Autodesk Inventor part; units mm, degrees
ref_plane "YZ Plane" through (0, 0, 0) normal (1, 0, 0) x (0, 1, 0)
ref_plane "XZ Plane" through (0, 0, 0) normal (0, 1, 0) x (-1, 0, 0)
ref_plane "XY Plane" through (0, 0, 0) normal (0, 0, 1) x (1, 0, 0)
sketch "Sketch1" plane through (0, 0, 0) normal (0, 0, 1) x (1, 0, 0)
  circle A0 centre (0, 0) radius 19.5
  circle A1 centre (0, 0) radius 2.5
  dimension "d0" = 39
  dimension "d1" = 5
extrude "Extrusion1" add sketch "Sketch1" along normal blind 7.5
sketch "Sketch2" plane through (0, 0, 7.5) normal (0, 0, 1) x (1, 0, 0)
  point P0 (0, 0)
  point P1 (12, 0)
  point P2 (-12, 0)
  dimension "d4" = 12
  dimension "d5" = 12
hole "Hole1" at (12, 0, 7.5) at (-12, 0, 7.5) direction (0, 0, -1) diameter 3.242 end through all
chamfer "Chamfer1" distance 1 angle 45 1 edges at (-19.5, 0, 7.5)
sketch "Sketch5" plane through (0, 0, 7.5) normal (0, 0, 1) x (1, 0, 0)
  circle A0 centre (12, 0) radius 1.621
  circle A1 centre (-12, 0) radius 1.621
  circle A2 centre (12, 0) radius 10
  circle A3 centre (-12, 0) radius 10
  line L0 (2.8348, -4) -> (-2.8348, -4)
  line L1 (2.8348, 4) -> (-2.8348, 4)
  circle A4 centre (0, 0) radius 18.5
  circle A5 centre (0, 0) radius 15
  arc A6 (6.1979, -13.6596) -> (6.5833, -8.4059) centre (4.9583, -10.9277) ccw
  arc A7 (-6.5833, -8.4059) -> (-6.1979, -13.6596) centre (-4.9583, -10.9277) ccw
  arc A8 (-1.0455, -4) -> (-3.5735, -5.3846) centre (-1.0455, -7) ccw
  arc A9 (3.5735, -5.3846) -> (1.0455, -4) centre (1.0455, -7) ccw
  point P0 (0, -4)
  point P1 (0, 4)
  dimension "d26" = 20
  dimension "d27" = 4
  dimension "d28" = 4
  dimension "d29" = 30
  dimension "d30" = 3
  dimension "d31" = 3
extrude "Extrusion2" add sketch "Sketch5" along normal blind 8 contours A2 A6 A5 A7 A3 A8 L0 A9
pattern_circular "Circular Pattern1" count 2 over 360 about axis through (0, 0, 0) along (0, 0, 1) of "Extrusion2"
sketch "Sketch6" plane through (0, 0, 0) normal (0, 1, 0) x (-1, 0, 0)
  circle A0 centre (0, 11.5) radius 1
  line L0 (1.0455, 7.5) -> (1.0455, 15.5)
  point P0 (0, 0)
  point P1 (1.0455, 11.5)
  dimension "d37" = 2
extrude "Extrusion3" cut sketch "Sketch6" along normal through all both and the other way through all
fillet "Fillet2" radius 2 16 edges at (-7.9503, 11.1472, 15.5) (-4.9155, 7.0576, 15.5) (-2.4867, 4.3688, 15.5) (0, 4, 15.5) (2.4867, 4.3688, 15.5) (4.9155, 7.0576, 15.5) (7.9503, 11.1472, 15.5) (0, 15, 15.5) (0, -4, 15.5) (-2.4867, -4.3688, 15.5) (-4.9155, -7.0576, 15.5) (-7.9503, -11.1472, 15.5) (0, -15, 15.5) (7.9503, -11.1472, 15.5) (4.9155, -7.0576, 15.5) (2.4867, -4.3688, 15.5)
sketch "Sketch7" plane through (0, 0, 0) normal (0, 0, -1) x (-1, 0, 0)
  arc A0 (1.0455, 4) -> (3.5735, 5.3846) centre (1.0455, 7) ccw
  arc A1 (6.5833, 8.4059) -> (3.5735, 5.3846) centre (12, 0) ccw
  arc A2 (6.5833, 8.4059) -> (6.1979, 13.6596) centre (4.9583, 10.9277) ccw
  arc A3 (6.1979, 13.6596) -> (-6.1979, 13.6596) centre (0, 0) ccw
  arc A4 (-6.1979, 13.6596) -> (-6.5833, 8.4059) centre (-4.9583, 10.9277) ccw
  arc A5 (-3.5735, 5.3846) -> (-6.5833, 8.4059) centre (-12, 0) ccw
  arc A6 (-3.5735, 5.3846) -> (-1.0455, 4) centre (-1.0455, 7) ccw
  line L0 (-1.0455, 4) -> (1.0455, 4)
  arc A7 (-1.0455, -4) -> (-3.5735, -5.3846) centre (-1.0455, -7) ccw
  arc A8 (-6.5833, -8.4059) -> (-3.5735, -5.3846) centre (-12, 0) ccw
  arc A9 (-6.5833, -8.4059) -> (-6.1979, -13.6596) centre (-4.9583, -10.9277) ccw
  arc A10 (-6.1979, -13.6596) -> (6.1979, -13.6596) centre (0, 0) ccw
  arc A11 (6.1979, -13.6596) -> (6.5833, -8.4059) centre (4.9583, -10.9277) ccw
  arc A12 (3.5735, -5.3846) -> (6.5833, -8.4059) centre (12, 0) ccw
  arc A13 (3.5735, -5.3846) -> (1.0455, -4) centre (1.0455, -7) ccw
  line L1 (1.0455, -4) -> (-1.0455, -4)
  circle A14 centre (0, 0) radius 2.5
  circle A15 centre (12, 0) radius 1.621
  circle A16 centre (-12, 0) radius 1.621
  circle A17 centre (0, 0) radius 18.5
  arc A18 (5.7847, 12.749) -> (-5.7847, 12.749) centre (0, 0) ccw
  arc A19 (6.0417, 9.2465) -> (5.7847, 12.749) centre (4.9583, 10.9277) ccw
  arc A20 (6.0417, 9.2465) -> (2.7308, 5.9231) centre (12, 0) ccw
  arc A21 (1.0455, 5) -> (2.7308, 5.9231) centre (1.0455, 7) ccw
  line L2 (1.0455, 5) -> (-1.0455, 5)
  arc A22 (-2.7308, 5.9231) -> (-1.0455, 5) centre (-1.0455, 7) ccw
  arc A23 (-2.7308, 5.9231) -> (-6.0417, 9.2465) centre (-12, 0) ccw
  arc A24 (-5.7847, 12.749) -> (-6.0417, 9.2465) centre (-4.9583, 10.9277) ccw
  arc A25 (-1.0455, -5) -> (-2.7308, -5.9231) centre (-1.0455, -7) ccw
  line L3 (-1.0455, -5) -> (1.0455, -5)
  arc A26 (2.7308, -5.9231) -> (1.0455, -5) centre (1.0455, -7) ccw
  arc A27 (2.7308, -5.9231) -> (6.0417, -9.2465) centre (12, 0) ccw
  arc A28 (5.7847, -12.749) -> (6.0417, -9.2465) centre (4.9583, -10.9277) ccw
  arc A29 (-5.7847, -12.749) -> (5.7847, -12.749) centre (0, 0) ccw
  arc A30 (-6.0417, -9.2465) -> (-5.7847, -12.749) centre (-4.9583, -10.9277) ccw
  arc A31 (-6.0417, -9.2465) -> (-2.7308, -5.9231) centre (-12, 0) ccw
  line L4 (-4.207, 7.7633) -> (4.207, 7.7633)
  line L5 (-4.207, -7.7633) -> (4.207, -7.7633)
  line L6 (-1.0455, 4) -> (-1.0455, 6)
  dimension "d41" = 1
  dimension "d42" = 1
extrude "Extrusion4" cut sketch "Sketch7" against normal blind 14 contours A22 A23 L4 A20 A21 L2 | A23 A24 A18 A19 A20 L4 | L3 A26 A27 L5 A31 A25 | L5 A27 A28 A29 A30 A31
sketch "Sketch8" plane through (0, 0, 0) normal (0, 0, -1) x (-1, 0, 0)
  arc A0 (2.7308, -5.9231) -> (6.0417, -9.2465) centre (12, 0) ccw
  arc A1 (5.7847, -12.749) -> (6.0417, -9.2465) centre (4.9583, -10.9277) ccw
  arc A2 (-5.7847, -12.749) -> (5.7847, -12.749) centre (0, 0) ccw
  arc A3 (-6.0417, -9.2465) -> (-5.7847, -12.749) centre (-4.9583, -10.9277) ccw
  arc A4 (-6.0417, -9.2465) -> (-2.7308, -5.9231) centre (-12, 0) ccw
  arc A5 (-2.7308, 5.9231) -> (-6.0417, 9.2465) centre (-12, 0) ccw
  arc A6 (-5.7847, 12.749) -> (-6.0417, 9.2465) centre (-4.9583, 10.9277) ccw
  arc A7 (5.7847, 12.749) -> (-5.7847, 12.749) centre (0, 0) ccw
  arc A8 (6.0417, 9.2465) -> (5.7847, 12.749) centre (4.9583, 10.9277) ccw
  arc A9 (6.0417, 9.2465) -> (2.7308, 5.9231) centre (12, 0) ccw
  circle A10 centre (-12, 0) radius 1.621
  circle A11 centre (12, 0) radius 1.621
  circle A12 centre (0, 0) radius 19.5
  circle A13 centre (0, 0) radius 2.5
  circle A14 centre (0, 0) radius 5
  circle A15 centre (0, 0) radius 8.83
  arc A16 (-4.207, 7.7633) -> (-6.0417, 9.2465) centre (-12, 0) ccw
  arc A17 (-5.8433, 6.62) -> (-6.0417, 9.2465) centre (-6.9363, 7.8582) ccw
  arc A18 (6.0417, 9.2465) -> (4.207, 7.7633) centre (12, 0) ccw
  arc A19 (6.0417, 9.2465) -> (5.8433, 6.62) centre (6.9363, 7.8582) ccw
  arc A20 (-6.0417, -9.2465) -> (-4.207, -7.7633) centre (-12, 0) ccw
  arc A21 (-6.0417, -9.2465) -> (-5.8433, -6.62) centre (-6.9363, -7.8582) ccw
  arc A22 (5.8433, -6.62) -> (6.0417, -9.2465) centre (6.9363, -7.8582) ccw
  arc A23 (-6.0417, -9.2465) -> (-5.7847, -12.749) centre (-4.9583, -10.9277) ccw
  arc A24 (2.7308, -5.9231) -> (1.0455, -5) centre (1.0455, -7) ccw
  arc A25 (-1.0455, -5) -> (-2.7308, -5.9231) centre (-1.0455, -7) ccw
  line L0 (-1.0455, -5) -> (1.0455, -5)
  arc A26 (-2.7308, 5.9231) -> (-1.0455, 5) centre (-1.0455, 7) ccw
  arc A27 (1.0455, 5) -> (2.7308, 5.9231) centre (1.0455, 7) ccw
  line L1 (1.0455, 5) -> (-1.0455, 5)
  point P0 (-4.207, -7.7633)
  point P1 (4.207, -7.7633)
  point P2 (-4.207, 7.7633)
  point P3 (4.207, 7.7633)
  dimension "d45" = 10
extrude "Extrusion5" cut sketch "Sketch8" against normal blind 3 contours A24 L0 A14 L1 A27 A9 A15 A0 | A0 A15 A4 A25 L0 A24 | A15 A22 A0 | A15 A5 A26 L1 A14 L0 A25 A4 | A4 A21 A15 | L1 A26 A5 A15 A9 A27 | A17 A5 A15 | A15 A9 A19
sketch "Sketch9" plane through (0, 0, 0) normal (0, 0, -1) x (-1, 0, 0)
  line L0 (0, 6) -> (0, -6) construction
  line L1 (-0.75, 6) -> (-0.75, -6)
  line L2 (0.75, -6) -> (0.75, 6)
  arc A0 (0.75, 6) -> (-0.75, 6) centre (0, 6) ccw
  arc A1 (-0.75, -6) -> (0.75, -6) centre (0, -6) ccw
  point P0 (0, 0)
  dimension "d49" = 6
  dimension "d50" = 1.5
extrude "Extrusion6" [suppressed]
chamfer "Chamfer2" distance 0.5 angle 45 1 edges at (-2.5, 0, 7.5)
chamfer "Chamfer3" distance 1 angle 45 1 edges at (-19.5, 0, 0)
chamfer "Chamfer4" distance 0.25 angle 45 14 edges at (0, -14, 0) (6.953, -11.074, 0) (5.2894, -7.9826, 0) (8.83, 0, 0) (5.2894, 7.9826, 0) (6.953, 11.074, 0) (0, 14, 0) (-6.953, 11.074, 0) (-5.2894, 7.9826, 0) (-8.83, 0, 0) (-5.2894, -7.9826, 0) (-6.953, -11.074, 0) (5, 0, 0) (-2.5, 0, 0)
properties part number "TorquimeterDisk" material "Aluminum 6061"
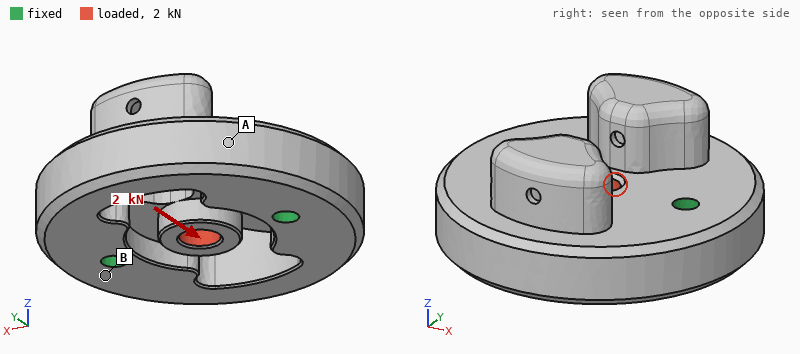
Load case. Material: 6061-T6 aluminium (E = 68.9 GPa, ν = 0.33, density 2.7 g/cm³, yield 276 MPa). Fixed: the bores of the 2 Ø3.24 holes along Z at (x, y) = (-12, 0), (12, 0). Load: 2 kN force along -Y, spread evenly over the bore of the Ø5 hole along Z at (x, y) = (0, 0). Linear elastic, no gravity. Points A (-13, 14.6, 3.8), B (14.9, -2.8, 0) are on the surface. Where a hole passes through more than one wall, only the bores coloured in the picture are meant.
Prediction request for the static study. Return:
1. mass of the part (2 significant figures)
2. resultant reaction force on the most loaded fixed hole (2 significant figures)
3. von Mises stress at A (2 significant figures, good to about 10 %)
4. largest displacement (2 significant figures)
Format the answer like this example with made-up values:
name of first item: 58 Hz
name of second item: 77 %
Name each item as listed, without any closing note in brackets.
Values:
mass of the part: 21 g
resultant reaction force on the most loaded fixed hole: 1.0 kN
von Mises stress at A: 10 MPa
largest displacement: 12 µm
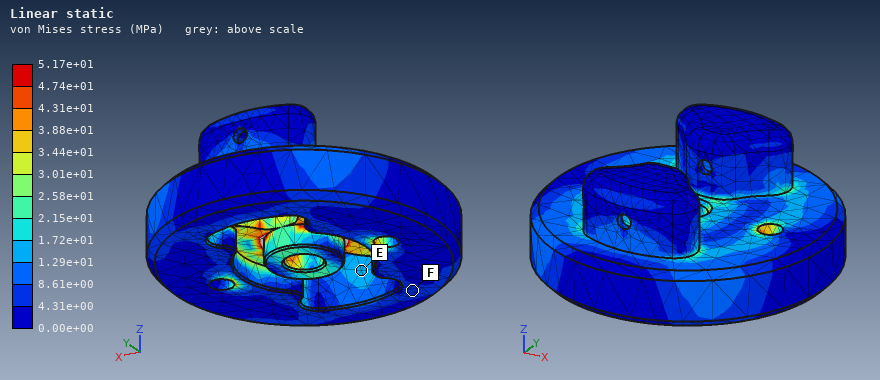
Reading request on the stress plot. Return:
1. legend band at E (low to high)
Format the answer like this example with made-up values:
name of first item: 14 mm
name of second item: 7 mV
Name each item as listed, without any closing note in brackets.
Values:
legend band at E: 1.29e+01 to 1.72e+01 MPa
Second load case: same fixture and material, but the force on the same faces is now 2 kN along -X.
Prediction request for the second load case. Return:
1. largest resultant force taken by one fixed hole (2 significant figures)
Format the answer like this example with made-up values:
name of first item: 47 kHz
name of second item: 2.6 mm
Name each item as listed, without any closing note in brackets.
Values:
largest resultant force taken by one fixed hole: 1.0 kN
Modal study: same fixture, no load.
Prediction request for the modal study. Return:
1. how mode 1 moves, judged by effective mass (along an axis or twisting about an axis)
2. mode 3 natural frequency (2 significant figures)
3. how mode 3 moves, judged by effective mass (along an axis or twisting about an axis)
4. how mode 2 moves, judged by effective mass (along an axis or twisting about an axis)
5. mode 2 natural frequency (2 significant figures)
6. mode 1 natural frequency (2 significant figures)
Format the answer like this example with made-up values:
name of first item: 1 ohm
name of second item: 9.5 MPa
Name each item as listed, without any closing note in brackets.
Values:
how mode 1 moves, judged by effective mass: twisting about X
mode 3 natural frequency: 22 kHz
how mode 3 moves, judged by effective mass: twisting about Z
how mode 2 moves, judged by effective mass: along Z
mode 2 natural frequency: 15 kHz
mode 1 natural frequency: 13 kHz
